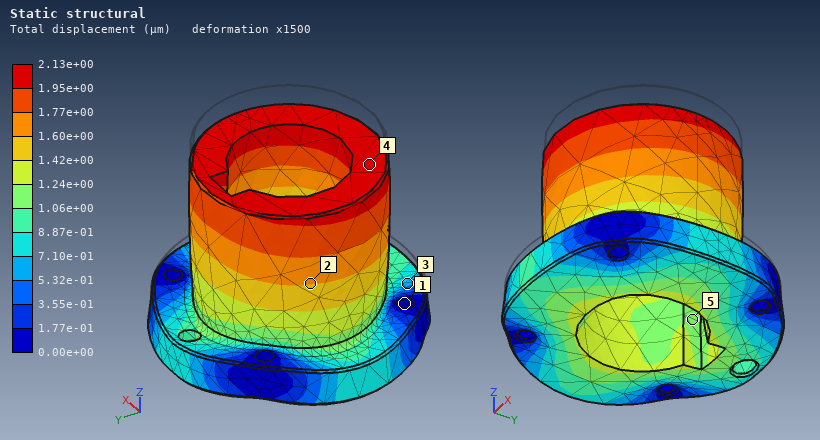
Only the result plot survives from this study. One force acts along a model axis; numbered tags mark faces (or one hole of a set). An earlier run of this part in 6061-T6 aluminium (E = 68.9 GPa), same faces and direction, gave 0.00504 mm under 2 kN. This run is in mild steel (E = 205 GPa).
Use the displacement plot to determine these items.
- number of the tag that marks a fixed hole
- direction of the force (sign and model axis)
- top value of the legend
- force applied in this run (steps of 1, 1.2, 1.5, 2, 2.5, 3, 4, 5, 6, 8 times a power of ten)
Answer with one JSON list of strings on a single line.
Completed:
["1", "-Z", "2.13e+00 µm", "2.5 kN"]
